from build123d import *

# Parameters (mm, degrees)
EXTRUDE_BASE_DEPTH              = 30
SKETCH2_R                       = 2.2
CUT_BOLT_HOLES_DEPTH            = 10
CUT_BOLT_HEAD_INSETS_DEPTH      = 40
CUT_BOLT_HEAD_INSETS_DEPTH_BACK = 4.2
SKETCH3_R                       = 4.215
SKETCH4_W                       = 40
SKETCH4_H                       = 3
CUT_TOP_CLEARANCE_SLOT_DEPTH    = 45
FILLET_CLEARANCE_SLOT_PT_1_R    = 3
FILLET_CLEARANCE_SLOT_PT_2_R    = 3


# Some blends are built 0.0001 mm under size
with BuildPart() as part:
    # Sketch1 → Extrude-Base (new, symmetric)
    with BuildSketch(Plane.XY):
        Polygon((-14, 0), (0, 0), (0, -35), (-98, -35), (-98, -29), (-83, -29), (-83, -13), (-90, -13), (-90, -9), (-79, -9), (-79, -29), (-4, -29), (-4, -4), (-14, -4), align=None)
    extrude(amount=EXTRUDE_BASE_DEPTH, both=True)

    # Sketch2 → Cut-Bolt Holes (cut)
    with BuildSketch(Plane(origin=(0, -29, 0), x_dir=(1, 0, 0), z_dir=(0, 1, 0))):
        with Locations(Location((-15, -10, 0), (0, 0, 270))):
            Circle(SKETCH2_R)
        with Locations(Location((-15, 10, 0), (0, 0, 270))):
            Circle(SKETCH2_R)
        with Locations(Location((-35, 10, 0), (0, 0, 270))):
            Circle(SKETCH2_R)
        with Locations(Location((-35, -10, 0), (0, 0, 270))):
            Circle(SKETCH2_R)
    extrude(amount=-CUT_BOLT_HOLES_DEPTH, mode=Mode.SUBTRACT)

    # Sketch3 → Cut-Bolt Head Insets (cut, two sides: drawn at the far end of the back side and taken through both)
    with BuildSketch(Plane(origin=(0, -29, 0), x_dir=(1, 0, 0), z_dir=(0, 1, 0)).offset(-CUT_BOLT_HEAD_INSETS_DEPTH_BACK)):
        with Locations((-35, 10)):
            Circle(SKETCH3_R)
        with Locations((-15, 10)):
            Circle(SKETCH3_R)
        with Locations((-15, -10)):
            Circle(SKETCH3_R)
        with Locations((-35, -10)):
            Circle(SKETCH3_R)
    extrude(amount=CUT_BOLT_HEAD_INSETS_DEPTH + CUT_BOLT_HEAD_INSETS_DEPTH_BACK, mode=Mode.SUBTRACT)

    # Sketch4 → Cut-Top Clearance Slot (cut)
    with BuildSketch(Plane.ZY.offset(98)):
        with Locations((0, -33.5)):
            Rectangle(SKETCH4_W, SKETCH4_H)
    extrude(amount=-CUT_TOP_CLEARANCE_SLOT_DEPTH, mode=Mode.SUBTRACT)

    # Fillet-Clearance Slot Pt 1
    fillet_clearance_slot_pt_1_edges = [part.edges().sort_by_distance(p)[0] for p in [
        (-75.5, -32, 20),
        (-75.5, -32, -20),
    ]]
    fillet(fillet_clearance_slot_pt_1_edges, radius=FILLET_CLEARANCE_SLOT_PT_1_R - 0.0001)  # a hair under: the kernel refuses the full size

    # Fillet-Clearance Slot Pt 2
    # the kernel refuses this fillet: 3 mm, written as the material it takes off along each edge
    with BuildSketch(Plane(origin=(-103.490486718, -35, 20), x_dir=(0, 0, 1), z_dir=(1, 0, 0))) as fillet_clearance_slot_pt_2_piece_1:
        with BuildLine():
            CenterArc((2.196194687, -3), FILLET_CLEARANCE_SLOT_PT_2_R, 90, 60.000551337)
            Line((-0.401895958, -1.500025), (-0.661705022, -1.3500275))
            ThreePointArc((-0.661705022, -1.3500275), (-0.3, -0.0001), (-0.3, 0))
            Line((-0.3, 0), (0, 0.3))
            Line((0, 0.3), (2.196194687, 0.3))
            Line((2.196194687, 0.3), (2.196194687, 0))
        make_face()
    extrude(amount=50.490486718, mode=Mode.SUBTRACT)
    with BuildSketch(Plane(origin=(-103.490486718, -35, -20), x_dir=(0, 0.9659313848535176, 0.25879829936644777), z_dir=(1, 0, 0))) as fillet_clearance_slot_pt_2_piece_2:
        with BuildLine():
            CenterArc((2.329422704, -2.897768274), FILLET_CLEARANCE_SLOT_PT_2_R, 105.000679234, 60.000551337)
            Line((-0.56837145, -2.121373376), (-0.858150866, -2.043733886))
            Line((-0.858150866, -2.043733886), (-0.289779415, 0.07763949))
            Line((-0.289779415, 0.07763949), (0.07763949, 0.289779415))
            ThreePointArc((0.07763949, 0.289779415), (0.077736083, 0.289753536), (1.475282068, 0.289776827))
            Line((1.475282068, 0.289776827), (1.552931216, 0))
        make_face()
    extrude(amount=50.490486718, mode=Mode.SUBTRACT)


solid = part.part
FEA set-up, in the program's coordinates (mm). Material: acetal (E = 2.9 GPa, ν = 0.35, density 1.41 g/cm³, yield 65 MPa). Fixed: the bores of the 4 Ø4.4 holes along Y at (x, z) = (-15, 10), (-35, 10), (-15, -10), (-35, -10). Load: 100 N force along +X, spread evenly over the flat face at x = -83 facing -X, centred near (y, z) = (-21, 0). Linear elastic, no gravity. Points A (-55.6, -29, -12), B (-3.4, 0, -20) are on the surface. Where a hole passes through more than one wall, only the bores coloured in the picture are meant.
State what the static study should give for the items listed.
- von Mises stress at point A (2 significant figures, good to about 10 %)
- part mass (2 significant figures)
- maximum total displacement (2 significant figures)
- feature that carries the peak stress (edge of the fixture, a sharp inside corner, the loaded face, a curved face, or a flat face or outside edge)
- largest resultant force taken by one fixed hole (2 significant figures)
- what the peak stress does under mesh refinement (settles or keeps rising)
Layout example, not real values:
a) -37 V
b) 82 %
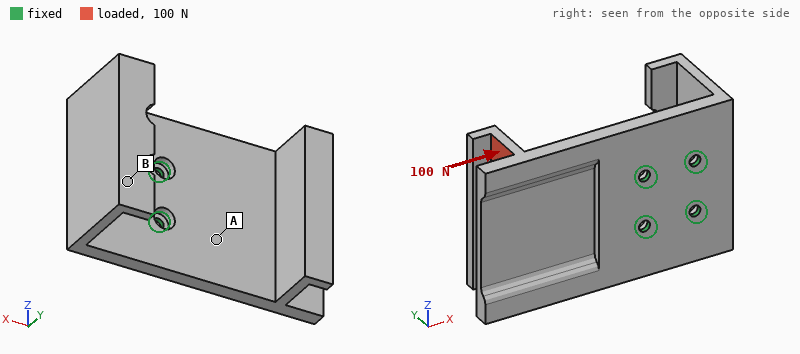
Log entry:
a) 4.5 MPa
b) 63 g
c) 1.2 mm
d) edge of the fixture
e) 56 N
f) keeps rising
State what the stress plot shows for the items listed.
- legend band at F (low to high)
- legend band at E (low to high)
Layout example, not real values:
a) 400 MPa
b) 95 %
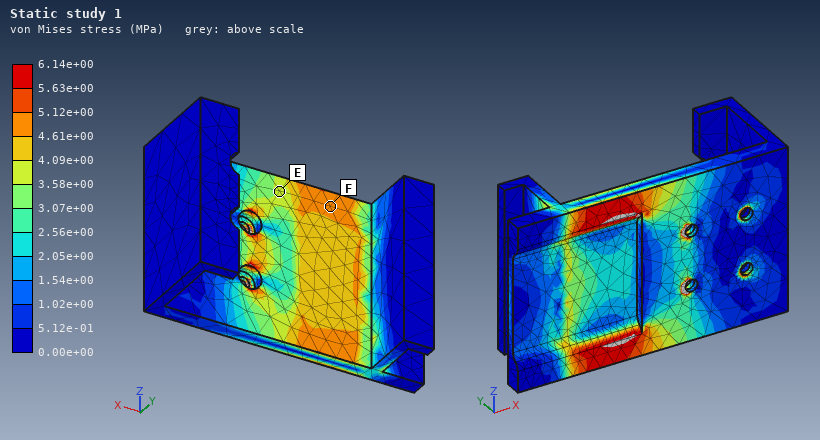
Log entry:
a) 4.61e+00 to 5.12e+00 MPa
b) 3.58e+00 to 4.09e+00 MPa
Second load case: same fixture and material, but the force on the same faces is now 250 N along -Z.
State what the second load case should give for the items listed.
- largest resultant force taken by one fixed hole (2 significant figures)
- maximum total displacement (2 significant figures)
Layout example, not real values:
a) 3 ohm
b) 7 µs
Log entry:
a) 370 N
b) 1.2 mm
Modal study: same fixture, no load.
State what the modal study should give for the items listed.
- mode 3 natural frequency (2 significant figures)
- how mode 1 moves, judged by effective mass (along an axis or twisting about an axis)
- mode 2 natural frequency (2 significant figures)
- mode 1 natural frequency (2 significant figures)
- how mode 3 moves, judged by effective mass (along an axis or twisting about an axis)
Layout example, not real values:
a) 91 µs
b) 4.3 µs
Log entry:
a) 520 Hz
b) along Y
c) 440 Hz
d) 230 Hz
e) along X
